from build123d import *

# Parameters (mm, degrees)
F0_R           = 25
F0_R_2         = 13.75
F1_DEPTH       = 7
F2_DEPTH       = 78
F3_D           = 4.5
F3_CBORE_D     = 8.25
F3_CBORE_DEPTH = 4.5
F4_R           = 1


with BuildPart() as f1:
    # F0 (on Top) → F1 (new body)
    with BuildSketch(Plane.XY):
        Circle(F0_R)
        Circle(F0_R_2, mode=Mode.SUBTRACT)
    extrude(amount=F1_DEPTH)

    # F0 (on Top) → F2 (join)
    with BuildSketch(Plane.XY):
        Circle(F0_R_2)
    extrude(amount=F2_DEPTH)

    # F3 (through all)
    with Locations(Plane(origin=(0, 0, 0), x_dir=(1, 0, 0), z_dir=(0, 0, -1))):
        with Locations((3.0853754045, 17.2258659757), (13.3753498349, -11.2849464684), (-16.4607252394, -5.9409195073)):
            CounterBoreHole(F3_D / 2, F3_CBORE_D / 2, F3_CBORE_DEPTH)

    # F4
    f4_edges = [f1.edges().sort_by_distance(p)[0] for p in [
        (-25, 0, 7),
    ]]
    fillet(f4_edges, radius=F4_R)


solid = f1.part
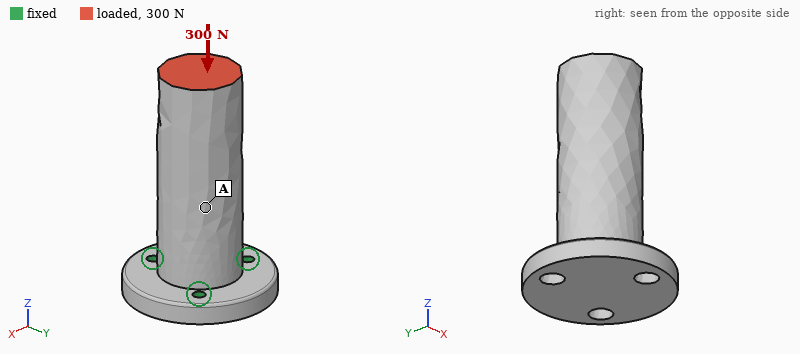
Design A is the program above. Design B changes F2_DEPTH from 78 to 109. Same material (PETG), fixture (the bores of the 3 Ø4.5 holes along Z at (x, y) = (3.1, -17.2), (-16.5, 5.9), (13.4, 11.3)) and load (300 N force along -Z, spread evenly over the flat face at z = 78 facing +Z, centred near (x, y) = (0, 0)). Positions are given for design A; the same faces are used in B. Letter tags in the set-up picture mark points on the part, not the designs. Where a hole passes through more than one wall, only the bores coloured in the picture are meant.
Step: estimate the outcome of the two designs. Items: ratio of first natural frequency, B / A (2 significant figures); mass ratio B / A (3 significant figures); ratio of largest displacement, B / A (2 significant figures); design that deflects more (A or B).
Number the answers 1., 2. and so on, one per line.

1. 0.55
2. 1.33
3. 1.2
4. B
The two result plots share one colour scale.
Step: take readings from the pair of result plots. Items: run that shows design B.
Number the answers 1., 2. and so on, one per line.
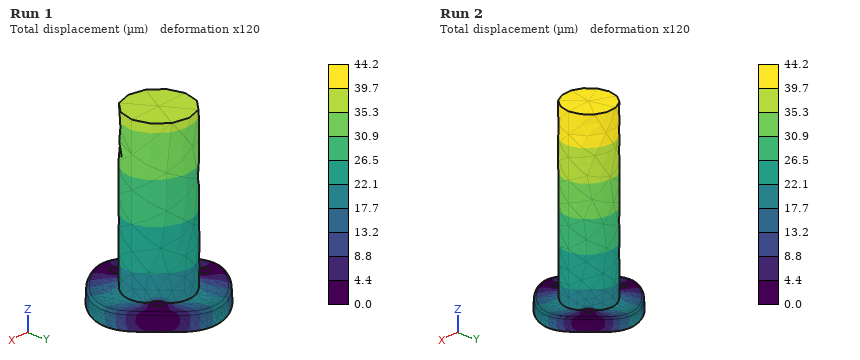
1. Run 2
